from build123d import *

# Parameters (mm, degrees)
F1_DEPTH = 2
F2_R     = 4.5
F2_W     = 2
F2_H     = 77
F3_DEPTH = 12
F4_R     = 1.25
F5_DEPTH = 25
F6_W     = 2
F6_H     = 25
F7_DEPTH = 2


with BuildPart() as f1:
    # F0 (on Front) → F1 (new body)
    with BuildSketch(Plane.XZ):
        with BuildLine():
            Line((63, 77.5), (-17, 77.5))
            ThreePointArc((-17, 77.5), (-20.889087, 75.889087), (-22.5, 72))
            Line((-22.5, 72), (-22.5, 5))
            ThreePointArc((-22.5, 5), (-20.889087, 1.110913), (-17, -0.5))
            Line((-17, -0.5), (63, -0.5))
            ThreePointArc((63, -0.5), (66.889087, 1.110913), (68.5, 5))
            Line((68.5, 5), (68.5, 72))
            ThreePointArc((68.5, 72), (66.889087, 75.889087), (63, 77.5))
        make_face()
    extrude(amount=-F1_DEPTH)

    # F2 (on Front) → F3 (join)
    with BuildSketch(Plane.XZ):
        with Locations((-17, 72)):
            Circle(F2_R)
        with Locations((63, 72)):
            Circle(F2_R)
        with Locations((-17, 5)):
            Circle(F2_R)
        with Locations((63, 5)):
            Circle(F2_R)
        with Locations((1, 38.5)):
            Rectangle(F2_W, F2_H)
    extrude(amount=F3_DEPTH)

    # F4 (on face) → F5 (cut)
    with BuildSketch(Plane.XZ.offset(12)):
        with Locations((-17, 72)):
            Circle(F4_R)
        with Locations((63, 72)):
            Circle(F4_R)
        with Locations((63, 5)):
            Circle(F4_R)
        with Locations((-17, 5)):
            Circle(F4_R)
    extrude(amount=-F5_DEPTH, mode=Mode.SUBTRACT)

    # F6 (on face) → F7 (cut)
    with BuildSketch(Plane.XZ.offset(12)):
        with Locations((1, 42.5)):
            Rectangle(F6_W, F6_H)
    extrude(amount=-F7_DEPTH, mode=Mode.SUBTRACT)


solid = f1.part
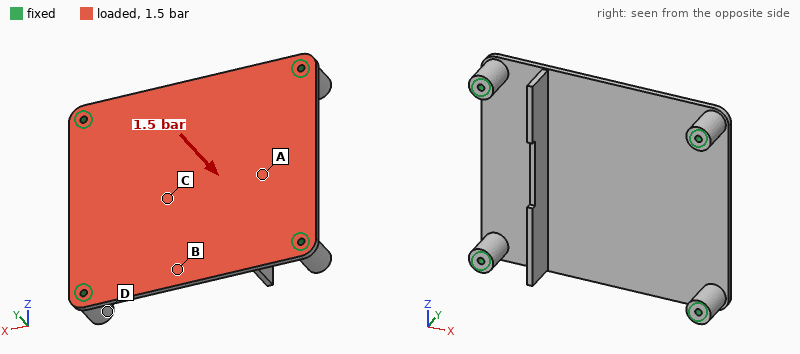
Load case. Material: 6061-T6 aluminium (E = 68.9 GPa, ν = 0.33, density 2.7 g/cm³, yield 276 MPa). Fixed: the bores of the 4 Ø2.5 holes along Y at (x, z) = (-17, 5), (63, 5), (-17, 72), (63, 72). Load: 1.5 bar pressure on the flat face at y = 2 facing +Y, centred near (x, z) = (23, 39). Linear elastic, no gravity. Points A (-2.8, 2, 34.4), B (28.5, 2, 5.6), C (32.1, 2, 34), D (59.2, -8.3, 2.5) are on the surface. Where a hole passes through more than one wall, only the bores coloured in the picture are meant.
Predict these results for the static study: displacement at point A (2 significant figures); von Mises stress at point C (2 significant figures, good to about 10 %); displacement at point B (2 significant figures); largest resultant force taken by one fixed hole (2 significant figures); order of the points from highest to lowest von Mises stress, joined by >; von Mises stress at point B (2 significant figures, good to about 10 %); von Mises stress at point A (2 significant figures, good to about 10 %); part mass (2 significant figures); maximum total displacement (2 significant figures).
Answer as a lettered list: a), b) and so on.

a) 0.19 mm
b) 52 MPa
c) 0.38 mm
d) 290 N
e) B > C > A > D
f) 65 MPa
g) 27 MPa
h) 50 g
i) 0.45 mm
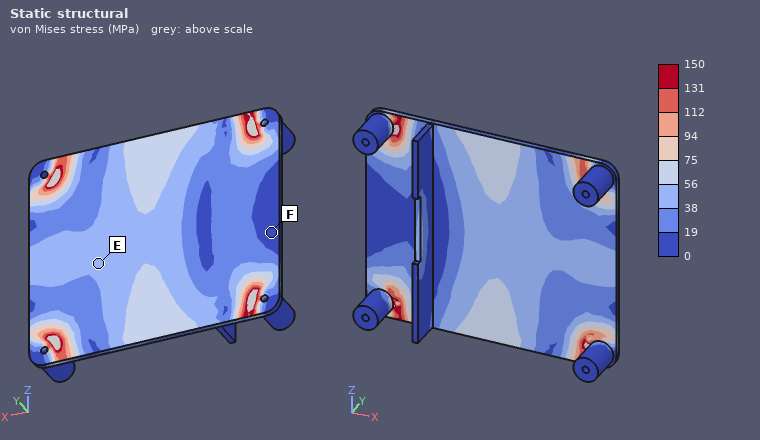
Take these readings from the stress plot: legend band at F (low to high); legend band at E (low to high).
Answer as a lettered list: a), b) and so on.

a) 0 to 19 MPa
b) 38 to 56 MPa
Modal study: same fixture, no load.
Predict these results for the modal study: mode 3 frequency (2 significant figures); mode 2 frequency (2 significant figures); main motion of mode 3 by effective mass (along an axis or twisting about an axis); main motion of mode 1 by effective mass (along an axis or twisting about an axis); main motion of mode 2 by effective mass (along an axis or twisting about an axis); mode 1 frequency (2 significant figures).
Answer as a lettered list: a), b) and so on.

a) 2700 Hz
b) 2100 Hz
c) twisting about Z
d) along Y
e) twisting about X
f) 1400 Hz
